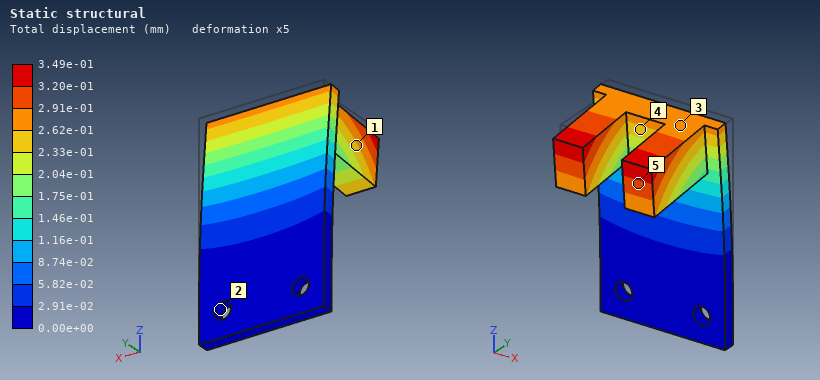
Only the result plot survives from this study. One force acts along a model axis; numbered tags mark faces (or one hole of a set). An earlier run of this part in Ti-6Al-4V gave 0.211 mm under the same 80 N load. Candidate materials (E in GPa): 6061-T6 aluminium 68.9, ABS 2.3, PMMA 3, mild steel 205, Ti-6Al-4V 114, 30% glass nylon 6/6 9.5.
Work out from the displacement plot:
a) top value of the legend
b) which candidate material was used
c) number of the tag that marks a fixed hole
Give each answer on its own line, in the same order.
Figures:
3.49e-01 mm
6061-T6 aluminium
2
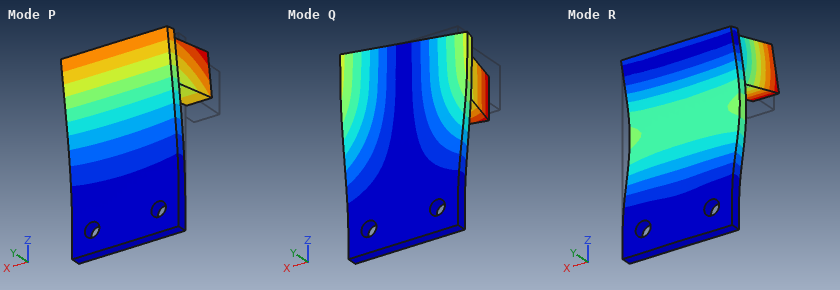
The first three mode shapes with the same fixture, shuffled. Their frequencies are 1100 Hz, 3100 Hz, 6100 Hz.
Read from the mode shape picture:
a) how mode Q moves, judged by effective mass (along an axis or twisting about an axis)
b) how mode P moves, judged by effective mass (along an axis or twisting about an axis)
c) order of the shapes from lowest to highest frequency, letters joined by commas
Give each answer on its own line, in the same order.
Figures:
along X
along Y
P, Q, R
